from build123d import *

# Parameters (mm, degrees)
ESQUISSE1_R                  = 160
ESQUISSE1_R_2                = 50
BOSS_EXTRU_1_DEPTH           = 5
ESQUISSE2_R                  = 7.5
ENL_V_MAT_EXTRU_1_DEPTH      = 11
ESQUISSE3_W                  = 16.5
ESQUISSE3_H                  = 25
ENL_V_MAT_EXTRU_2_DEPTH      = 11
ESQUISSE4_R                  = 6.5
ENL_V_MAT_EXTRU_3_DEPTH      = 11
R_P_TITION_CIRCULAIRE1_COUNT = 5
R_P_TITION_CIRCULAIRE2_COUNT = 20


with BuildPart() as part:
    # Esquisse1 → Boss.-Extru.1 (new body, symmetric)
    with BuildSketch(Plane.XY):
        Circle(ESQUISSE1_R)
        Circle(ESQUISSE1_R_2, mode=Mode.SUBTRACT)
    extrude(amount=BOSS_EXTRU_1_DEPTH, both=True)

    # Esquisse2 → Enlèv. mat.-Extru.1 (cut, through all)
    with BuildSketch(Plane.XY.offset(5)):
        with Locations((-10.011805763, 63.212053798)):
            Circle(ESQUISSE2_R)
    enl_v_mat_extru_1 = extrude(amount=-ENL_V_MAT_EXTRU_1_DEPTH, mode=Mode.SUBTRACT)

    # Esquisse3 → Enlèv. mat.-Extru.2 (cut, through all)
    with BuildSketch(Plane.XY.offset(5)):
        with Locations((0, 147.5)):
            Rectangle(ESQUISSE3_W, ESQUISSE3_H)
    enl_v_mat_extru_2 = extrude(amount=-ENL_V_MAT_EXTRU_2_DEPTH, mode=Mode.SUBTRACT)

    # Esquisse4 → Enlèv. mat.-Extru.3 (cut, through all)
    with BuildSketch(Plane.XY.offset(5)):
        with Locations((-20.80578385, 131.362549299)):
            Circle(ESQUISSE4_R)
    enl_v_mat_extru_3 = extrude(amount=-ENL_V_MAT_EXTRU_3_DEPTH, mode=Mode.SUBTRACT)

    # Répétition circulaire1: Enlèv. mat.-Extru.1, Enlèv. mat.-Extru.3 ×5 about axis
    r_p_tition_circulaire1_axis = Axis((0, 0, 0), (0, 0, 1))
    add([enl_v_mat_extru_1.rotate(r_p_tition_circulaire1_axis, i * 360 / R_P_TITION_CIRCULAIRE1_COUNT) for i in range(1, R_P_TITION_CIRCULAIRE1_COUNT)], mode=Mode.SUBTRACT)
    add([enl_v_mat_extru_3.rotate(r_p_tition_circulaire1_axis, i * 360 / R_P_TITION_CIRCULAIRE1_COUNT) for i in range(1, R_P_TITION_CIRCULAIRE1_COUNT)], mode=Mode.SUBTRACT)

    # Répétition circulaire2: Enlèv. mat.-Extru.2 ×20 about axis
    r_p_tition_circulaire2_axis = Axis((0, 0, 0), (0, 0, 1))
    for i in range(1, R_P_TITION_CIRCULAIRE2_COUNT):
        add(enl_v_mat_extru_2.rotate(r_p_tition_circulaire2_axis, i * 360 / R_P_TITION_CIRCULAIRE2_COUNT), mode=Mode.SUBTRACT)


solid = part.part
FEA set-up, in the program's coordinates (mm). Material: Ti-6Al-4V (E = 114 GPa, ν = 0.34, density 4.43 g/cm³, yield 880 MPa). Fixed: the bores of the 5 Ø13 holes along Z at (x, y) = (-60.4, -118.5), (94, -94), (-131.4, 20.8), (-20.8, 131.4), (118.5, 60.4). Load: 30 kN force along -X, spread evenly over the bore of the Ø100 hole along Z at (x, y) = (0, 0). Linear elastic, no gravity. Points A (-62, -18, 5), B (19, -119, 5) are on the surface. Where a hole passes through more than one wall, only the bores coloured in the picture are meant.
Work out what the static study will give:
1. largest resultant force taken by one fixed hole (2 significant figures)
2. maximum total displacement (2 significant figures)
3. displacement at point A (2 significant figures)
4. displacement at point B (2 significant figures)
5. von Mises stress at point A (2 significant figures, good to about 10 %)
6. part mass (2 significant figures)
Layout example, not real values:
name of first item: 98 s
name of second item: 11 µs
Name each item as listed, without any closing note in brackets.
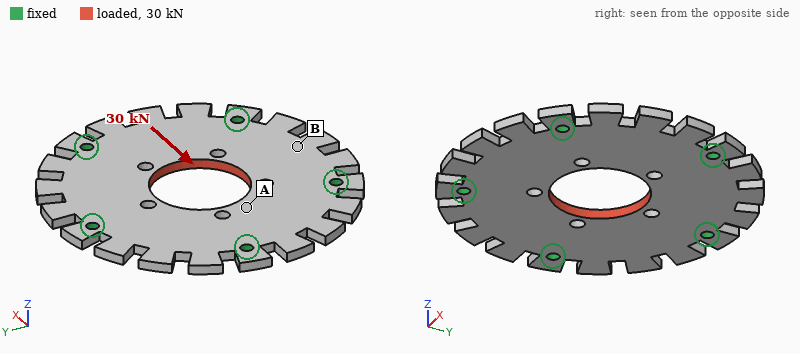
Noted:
largest resultant force taken by one fixed hole: 8.3 kN
maximum total displacement: 15 µm
displacement at point A: 12 µm
displacement at point B: 3.5 µm
von Mises stress at point A: 9.8 MPa
part mass: 2.8 kg
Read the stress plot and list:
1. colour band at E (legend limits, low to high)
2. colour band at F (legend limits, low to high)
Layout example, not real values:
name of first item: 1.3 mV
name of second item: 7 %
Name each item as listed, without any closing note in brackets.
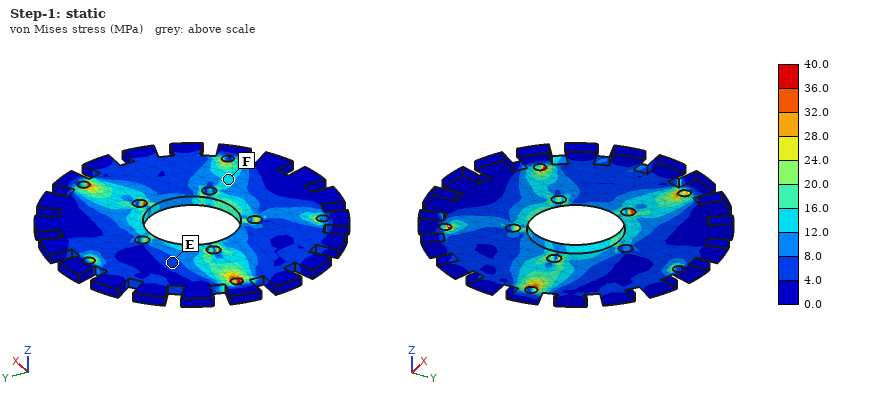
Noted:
colour band at E: 4.0 to 8.0 MPa
colour band at F: 12.0 to 16.0 MPa
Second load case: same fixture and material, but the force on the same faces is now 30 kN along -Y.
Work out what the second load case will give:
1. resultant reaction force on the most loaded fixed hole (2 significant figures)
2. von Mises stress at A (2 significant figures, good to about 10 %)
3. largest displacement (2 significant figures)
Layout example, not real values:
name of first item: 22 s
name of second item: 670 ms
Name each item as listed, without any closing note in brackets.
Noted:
resultant reaction force on the most loaded fixed hole: 8.3 kN
von Mises stress at A: 11 MPa
largest displacement: 15 µm
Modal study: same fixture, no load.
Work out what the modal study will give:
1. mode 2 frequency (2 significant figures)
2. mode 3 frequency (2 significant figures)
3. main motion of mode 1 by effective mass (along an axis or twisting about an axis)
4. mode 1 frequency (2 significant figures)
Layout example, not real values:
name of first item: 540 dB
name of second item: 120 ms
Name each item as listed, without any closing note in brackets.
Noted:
mode 2 frequency: 1500 Hz
mode 3 frequency: 1500 Hz
main motion of mode 1 by effective mass: along Z
mode 1 frequency: 1200 Hz
